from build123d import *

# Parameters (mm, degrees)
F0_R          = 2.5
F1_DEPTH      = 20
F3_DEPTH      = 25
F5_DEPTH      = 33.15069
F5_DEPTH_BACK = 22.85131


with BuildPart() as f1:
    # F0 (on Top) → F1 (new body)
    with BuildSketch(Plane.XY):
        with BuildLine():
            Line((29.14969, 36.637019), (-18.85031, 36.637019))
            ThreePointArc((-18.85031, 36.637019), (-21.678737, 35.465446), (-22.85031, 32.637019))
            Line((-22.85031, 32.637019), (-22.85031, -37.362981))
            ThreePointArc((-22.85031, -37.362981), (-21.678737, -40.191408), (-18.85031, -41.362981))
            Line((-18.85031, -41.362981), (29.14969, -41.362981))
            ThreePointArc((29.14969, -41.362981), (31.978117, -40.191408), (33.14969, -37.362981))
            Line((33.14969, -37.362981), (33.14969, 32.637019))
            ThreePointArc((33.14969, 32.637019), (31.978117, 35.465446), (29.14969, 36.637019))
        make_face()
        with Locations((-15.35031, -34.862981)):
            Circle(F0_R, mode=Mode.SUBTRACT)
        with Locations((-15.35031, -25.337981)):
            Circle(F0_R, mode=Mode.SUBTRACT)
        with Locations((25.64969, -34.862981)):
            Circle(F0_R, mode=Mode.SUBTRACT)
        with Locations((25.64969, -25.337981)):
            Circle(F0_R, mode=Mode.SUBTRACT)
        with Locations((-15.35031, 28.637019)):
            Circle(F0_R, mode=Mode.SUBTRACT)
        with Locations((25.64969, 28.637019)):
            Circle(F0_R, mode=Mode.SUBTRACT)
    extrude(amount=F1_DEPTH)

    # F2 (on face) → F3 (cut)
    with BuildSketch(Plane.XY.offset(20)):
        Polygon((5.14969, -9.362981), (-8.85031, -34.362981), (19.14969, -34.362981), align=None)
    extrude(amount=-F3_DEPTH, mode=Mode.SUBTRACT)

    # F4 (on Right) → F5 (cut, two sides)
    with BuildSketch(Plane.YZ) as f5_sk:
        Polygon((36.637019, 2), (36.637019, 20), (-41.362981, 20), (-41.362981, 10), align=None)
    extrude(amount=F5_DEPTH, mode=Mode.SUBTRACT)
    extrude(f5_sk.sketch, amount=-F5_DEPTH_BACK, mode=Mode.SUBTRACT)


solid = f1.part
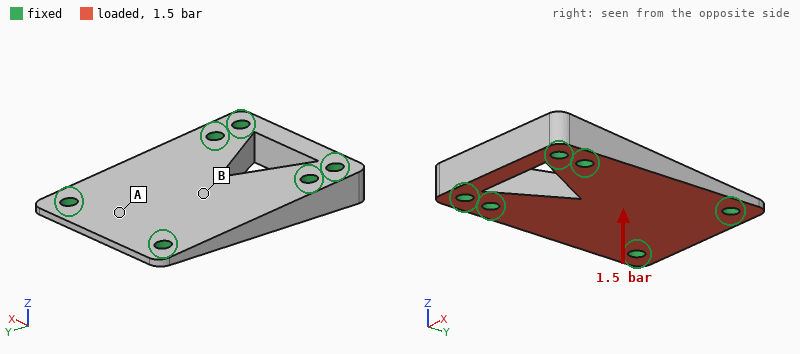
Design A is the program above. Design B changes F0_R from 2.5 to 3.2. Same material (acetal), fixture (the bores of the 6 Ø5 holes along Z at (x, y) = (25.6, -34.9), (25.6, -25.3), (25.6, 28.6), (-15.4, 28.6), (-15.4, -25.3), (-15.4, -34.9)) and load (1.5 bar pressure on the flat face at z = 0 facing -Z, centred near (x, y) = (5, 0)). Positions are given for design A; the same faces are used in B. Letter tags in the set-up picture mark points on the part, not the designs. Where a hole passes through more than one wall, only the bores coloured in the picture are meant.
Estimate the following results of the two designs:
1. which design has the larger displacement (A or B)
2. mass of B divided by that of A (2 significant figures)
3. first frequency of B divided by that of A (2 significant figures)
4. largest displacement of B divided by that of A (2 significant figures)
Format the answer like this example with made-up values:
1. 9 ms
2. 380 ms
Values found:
1. A
2. 0.98
3. 1.1
4. 0.86
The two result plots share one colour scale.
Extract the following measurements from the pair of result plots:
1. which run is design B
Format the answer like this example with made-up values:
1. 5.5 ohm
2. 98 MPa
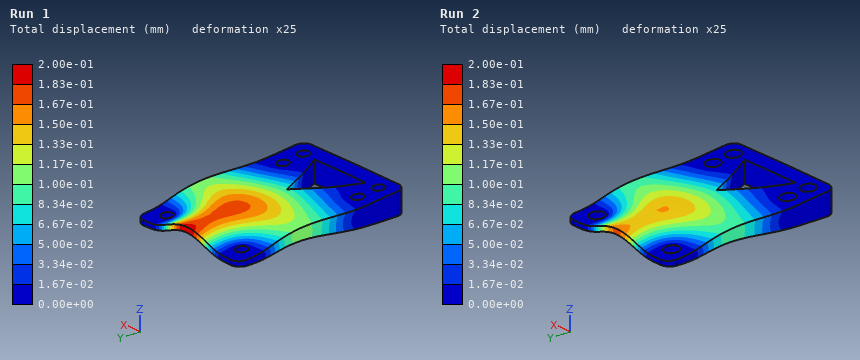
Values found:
1. Run 2
